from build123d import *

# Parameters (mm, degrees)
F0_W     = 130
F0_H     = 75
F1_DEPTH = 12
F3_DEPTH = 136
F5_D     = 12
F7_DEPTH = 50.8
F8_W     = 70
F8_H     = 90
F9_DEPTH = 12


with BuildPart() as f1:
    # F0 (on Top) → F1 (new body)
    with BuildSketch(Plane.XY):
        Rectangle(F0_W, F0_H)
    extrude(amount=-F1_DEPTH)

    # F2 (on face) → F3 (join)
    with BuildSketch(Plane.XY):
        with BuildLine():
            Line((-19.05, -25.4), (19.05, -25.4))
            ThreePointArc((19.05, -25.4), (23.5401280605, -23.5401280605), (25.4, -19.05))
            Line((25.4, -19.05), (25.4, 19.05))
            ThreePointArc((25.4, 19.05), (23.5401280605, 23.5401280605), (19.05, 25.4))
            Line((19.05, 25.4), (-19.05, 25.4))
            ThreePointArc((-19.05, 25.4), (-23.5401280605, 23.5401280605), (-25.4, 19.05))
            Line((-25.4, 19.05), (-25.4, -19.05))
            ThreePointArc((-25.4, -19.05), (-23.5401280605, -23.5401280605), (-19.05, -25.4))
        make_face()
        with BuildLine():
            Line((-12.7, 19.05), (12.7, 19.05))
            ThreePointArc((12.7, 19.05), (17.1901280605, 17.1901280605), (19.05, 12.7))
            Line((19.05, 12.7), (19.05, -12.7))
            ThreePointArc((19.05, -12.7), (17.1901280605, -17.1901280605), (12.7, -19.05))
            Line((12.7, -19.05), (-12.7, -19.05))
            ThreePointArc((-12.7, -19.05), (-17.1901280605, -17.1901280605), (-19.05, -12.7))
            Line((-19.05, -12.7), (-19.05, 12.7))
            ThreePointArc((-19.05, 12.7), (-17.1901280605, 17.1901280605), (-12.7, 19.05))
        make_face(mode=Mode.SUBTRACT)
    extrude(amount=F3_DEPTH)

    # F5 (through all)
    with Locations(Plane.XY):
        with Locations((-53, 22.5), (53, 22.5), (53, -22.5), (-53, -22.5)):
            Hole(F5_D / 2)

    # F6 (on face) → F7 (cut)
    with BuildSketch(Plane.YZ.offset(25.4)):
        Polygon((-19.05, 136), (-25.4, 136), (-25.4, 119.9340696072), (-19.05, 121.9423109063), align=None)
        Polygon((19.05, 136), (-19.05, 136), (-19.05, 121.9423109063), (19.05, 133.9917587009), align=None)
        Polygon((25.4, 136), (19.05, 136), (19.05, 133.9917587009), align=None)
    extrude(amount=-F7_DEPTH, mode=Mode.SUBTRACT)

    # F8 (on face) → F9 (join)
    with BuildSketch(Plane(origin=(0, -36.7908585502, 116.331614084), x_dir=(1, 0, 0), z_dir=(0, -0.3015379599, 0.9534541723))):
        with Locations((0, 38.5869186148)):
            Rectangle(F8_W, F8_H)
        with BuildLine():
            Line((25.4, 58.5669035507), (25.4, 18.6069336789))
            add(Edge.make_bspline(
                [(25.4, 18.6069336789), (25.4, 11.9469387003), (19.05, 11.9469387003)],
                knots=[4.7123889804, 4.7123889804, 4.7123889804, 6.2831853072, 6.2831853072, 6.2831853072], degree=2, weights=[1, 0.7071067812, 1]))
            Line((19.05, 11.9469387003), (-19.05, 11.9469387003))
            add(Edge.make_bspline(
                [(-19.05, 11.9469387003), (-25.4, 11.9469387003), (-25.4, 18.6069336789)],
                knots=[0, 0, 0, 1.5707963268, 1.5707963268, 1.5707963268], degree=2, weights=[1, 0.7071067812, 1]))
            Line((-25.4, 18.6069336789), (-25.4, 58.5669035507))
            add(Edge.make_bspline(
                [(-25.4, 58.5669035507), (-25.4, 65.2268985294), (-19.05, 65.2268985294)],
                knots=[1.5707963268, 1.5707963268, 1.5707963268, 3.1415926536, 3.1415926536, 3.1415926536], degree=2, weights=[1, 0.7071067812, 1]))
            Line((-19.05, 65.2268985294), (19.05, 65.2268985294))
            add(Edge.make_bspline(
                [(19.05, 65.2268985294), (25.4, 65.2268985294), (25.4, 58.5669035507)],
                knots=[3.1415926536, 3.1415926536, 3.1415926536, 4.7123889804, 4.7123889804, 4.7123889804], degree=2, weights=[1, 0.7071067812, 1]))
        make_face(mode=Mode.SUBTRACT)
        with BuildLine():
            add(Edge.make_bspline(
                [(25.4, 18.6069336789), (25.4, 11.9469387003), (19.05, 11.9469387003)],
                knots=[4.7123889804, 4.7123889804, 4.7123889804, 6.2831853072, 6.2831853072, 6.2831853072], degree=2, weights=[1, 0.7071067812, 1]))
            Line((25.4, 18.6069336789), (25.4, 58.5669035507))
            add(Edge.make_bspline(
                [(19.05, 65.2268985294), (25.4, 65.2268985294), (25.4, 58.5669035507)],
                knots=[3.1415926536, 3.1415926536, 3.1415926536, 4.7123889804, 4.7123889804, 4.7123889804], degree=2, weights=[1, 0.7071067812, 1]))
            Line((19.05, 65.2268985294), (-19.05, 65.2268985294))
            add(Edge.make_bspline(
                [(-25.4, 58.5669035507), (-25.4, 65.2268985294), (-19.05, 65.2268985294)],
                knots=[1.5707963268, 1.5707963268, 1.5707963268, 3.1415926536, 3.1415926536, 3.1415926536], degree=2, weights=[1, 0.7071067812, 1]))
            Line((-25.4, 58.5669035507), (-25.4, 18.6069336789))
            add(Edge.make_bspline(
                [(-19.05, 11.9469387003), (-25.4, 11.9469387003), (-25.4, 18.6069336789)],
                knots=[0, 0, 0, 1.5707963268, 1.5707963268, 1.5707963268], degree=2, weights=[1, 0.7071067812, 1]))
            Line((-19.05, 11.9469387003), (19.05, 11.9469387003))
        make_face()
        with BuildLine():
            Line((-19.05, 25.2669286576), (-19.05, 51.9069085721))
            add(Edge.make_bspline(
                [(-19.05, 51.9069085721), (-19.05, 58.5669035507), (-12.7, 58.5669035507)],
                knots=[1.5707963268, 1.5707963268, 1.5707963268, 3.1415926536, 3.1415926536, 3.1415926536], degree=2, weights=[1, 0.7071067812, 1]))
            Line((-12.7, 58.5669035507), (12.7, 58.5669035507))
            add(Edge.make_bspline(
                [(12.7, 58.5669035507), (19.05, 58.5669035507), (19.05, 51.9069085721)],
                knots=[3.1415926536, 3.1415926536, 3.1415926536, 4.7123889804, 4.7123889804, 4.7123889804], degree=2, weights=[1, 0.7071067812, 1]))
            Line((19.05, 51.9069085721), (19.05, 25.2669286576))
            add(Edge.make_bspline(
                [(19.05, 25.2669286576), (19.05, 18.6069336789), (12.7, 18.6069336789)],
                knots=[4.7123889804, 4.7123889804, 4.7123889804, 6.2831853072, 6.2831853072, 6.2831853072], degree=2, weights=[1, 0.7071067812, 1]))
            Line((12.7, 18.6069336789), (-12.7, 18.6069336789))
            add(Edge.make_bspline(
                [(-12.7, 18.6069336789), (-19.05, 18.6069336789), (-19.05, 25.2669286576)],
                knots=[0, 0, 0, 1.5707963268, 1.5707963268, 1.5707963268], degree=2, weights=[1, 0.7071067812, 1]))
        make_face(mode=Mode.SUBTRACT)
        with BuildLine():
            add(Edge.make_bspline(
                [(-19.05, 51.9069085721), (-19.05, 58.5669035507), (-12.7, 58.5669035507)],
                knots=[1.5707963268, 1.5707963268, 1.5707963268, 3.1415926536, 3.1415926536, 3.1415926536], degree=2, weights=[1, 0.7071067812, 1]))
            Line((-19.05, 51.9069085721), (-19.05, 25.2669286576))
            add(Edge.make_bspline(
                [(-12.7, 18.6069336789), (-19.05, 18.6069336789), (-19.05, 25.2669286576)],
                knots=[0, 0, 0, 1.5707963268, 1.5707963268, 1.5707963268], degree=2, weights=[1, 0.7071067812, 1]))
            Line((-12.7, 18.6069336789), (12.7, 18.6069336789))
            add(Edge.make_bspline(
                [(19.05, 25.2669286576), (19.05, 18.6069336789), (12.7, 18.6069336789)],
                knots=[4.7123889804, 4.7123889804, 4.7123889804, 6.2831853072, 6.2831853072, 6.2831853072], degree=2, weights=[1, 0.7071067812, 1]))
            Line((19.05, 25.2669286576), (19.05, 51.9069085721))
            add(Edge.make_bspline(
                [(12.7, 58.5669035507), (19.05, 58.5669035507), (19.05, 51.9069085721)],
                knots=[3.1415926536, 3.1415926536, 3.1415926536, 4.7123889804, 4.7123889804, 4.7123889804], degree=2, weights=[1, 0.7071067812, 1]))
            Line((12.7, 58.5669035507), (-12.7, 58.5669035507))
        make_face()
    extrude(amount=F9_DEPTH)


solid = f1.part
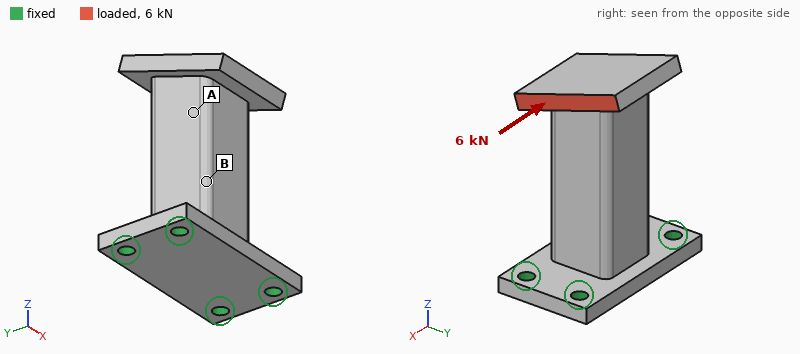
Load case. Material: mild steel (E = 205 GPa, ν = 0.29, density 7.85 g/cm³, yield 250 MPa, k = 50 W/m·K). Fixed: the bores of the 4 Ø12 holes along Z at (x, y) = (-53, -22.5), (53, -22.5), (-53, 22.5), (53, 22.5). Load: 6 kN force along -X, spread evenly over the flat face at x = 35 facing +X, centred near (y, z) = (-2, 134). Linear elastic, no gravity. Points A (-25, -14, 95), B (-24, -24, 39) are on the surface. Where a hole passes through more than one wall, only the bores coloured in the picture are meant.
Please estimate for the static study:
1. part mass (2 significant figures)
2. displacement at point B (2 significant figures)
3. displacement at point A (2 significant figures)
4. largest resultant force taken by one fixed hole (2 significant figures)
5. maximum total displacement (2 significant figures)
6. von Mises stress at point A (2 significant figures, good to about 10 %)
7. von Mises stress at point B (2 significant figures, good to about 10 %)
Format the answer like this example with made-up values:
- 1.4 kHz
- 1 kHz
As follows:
- 2.6 kg
- 0.045 mm
- 0.11 mm
- 5.7 kN
- 0.19 mm
- 17 MPa
- 35 MPa
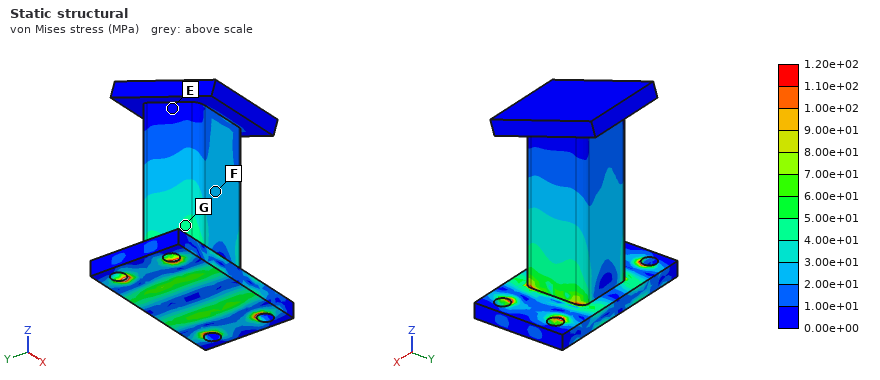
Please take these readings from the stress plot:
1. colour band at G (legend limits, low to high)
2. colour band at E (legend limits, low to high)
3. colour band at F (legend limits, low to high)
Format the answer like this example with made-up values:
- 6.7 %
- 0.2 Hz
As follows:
- 4.00e+01 to 5.00e+01 MPa
- 0.00e+00 to 1.00e+01 MPa
- 2.00e+01 to 3.00e+01 MPa
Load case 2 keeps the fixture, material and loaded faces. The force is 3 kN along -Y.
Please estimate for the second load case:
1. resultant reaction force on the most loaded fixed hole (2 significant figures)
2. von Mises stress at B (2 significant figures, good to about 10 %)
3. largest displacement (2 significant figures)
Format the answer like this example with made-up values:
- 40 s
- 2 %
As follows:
- 4.4 kN
- 17 MPa
- 0.18 mm
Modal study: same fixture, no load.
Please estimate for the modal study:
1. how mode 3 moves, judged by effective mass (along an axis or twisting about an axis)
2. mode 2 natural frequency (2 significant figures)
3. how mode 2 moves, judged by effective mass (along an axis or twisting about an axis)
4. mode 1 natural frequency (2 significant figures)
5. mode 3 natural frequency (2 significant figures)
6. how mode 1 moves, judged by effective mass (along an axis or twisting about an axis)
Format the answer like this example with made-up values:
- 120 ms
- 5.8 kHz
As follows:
- along Z
- 1000 Hz
- along X
- 730 Hz
- 3000 Hz
- along Y
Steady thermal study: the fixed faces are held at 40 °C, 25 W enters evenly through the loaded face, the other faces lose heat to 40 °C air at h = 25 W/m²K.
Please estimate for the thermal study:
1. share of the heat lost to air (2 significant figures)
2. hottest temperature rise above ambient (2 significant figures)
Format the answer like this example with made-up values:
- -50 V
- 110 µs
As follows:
- 80 %
- 35 K
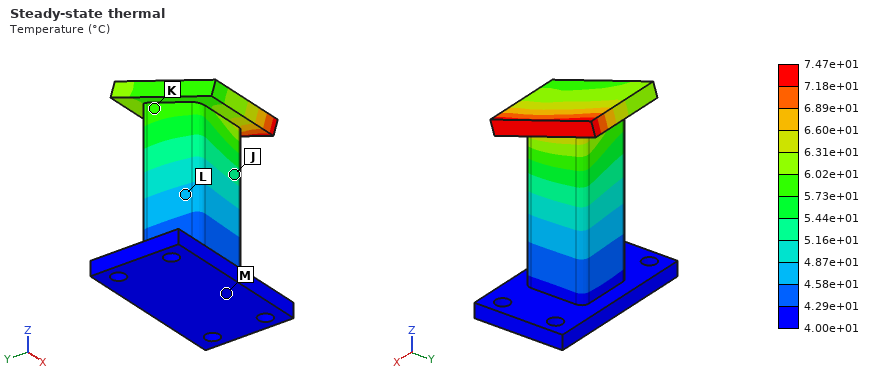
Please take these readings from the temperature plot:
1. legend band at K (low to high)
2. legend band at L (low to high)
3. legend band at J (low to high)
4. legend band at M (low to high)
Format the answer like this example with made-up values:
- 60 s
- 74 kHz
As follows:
- 5.73e+01 to 6.02e+01 °C
- 4.58e+01 to 4.87e+01 °C
- 5.16e+01 to 5.44e+01 °C
- 4.00e+01 to 4.29e+01 °C
